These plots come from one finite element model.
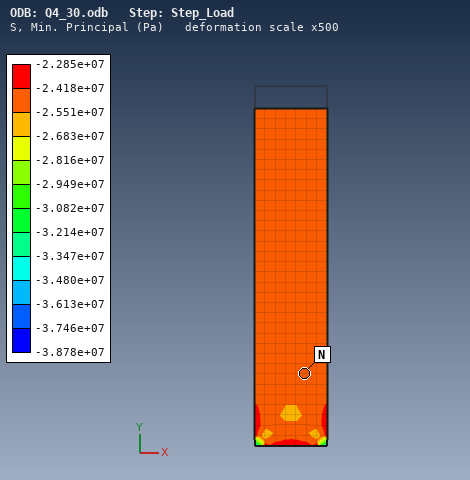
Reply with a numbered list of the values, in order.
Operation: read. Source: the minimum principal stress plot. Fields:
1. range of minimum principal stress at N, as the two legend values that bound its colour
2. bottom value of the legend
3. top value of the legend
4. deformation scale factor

1. -2.551e+07 to -2.418e+07 Pa
2. -3.878e+07 Pa
3. -2.285e+07 Pa
4. 500
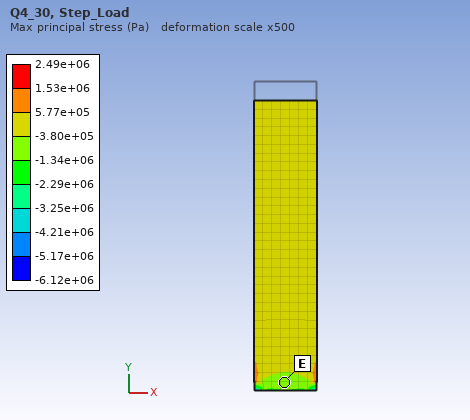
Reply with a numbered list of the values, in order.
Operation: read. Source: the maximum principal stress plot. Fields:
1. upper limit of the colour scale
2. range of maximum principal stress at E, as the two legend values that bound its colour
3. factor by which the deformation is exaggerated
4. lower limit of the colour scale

1. 2.49e+06 Pa
2. -1.34e+06 to -3.80e+05 Pa
3. 500
4. -6.12e+06 Pa
